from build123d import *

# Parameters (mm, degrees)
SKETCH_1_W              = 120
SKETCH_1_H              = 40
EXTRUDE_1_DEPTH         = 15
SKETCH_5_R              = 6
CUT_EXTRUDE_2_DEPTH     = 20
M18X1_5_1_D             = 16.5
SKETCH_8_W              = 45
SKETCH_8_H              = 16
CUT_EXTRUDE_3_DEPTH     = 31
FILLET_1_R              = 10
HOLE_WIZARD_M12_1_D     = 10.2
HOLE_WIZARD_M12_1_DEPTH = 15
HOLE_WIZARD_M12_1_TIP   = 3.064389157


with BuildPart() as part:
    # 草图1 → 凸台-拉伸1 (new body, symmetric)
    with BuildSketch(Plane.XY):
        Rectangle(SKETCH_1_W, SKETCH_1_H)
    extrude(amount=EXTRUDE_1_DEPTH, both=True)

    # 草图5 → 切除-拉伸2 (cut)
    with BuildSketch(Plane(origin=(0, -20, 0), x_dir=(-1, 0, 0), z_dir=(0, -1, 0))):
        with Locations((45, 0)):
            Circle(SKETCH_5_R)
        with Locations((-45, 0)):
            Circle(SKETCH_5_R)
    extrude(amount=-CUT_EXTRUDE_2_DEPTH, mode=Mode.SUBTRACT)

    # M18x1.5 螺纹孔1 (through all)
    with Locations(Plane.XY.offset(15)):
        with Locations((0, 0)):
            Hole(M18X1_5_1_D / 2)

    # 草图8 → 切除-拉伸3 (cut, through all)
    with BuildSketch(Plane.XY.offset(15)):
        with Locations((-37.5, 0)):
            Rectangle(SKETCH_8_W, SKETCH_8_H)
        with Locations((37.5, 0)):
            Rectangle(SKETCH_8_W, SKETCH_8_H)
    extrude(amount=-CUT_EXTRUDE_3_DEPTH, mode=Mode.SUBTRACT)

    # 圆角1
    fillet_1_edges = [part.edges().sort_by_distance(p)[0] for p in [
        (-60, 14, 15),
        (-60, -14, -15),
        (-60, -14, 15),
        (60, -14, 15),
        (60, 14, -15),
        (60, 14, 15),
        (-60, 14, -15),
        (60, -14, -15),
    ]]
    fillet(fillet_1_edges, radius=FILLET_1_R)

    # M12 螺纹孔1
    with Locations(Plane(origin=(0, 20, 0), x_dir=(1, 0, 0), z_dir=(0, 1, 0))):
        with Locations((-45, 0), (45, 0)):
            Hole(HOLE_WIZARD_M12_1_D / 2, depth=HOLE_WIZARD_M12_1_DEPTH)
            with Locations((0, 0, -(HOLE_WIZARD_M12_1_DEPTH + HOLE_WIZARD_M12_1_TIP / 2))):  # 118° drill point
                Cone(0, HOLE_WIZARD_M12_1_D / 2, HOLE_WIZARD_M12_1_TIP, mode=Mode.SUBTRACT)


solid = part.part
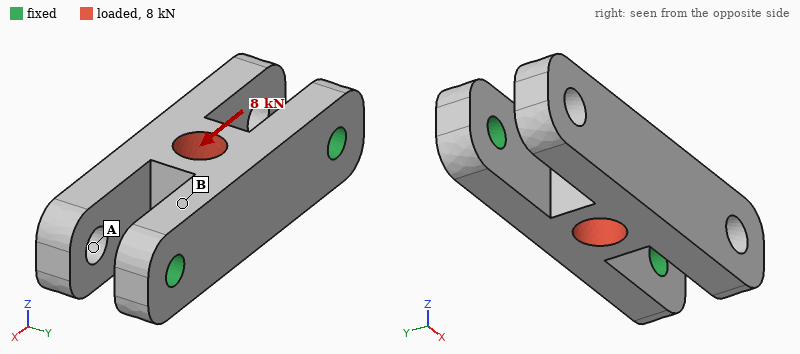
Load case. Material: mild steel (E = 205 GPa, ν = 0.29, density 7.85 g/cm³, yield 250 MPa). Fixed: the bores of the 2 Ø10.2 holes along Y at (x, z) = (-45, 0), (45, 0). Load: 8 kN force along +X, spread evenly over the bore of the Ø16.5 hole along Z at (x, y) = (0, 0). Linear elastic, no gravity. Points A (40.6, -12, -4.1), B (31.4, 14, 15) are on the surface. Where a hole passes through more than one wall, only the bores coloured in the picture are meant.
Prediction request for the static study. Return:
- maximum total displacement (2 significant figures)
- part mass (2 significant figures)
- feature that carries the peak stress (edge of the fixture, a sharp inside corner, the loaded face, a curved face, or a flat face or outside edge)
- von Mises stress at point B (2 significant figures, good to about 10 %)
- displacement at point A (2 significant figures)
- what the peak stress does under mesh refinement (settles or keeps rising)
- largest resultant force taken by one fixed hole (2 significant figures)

25 µm
690 g
edge of the fixture
15 MPa
19 µm
keeps rising
4.4 kN
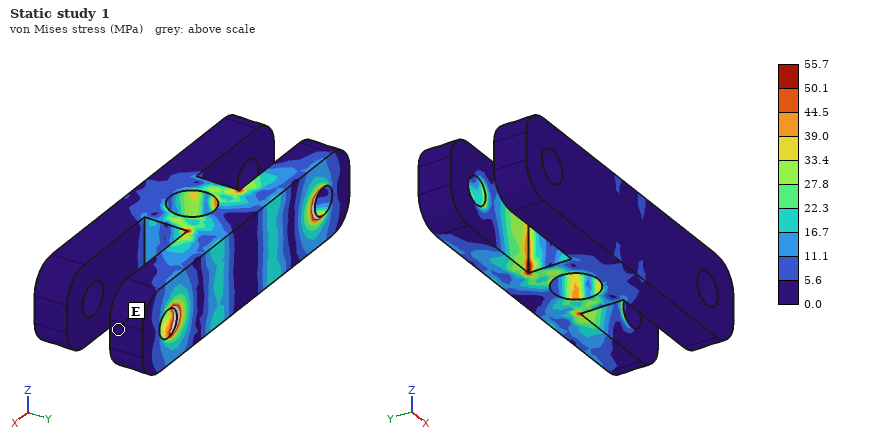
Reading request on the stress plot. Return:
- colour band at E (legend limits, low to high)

0.0 to 5.6 MPa
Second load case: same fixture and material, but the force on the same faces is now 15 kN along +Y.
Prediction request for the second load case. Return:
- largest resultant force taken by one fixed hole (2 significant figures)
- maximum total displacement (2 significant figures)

7.7 kN
49 µm
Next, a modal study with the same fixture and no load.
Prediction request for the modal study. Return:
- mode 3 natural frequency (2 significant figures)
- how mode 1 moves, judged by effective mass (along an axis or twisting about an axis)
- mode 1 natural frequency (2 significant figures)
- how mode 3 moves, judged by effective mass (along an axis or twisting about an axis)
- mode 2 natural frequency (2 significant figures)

3100 Hz
along Z
2200 Hz
along Y
2700 Hz
